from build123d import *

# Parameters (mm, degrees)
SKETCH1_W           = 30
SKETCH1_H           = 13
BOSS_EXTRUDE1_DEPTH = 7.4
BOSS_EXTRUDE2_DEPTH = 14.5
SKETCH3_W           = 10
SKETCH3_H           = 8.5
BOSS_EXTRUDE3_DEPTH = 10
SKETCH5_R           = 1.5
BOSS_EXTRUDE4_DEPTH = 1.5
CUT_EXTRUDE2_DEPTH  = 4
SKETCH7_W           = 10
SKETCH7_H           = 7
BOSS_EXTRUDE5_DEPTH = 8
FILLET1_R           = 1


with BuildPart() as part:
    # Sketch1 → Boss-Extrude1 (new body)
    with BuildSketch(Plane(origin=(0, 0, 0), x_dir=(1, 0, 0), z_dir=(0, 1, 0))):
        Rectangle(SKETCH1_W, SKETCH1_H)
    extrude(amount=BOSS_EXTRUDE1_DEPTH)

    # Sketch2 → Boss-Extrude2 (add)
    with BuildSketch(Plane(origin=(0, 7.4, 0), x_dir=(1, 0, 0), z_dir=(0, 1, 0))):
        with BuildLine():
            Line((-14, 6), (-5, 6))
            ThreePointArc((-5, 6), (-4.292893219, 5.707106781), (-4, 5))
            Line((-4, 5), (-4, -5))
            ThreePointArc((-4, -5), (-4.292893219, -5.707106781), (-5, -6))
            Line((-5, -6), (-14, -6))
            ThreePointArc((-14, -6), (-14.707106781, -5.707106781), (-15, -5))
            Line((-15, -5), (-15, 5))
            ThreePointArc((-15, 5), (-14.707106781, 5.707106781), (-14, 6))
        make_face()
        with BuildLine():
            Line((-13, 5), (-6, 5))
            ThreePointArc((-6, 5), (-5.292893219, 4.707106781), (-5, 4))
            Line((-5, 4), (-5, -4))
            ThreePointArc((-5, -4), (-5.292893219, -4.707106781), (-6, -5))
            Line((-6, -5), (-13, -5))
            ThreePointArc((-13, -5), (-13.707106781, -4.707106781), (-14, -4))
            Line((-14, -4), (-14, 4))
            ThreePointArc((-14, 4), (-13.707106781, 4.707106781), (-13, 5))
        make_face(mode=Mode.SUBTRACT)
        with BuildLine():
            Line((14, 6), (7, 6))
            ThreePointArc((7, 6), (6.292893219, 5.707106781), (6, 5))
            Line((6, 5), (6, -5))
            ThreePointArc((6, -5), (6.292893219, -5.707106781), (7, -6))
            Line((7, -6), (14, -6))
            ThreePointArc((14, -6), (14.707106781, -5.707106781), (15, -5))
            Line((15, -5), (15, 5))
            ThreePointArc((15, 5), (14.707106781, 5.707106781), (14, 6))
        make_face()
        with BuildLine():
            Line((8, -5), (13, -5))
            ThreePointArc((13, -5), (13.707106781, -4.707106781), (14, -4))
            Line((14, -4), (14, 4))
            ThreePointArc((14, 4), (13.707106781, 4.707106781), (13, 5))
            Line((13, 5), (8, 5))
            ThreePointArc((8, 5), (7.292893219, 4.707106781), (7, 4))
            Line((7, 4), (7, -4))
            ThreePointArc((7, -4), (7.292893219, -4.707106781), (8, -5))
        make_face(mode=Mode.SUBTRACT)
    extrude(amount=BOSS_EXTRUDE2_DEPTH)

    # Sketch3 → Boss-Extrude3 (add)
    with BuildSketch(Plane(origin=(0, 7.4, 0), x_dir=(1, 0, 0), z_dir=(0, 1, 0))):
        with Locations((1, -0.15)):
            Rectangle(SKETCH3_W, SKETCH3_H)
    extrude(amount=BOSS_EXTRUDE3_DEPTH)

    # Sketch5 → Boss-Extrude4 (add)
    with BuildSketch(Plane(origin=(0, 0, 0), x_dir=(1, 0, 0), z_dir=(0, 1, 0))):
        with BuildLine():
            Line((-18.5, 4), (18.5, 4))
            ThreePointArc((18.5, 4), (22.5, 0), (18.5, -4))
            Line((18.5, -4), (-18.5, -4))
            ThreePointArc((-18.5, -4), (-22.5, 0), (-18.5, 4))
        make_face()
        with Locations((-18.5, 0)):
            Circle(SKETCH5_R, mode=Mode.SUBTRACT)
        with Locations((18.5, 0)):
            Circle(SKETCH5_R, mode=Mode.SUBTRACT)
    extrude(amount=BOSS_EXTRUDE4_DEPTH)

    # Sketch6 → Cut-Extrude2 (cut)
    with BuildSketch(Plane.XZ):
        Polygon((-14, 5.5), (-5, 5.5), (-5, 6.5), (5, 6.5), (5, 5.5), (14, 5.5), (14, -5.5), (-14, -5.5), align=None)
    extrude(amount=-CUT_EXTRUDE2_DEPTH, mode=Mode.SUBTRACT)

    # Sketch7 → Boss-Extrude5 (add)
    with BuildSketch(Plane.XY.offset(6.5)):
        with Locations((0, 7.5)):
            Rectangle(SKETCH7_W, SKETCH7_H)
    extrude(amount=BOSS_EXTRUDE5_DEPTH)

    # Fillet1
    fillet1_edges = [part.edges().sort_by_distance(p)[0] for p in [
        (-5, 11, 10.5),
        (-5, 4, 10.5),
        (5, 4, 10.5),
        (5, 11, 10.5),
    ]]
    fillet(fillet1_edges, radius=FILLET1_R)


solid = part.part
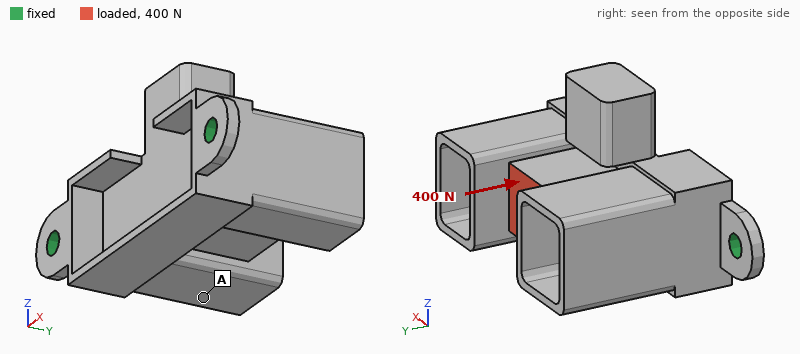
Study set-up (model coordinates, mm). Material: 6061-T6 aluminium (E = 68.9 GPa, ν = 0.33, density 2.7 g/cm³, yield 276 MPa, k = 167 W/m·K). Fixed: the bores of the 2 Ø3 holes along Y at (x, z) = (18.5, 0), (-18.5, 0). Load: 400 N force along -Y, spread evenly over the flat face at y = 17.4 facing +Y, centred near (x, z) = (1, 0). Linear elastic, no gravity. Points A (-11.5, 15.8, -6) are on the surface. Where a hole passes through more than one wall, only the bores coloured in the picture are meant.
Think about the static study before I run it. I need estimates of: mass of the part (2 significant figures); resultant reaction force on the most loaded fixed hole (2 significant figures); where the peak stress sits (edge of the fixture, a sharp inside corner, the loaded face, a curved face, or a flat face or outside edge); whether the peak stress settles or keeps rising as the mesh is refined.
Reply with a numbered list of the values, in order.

1. 12 g
2. 240 N
3. edge of the fixture
4. keeps rising
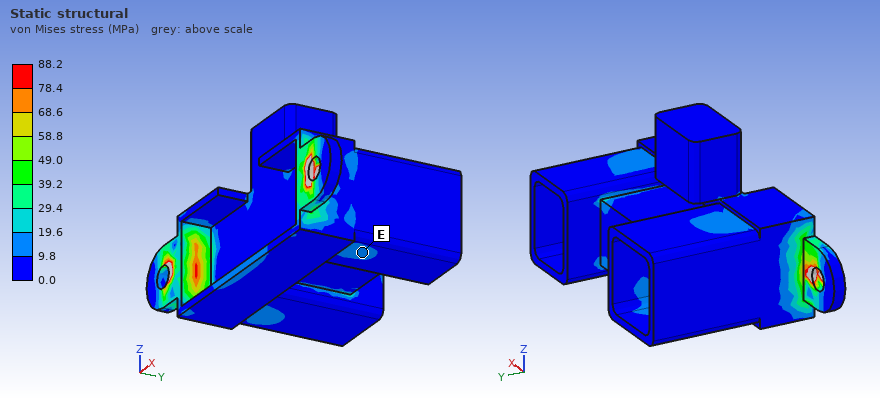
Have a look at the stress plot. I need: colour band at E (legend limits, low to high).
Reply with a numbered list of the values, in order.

1. 9.8 to 19.6 MPa
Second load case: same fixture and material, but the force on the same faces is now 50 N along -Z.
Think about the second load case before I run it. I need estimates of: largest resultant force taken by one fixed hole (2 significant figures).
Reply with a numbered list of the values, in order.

1. 26 N
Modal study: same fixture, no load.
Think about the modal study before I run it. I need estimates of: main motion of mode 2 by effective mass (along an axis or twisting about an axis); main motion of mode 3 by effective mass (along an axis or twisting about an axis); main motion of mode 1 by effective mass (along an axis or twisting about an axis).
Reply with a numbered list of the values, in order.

1. along Y
2. along X
3. along Z
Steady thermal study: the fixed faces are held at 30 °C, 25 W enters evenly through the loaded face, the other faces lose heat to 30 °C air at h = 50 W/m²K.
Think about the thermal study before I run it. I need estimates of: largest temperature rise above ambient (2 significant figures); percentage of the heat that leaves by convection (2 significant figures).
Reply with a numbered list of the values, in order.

1. 49 K
2. 29 %
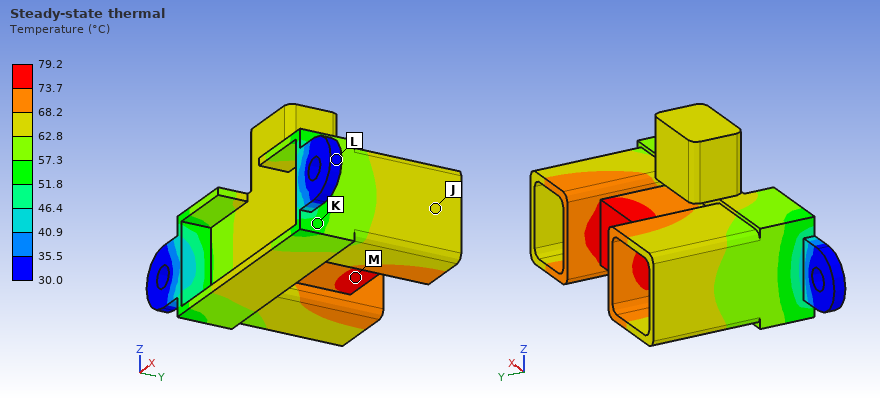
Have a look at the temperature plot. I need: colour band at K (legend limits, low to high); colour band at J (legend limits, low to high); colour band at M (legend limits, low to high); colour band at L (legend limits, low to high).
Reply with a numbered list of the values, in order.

1. 51.8 to 57.3 °C
2. 62.8 to 68.2 °C
3. 73.7 to 79.2 °C
4. 30.0 to 35.5 °C
